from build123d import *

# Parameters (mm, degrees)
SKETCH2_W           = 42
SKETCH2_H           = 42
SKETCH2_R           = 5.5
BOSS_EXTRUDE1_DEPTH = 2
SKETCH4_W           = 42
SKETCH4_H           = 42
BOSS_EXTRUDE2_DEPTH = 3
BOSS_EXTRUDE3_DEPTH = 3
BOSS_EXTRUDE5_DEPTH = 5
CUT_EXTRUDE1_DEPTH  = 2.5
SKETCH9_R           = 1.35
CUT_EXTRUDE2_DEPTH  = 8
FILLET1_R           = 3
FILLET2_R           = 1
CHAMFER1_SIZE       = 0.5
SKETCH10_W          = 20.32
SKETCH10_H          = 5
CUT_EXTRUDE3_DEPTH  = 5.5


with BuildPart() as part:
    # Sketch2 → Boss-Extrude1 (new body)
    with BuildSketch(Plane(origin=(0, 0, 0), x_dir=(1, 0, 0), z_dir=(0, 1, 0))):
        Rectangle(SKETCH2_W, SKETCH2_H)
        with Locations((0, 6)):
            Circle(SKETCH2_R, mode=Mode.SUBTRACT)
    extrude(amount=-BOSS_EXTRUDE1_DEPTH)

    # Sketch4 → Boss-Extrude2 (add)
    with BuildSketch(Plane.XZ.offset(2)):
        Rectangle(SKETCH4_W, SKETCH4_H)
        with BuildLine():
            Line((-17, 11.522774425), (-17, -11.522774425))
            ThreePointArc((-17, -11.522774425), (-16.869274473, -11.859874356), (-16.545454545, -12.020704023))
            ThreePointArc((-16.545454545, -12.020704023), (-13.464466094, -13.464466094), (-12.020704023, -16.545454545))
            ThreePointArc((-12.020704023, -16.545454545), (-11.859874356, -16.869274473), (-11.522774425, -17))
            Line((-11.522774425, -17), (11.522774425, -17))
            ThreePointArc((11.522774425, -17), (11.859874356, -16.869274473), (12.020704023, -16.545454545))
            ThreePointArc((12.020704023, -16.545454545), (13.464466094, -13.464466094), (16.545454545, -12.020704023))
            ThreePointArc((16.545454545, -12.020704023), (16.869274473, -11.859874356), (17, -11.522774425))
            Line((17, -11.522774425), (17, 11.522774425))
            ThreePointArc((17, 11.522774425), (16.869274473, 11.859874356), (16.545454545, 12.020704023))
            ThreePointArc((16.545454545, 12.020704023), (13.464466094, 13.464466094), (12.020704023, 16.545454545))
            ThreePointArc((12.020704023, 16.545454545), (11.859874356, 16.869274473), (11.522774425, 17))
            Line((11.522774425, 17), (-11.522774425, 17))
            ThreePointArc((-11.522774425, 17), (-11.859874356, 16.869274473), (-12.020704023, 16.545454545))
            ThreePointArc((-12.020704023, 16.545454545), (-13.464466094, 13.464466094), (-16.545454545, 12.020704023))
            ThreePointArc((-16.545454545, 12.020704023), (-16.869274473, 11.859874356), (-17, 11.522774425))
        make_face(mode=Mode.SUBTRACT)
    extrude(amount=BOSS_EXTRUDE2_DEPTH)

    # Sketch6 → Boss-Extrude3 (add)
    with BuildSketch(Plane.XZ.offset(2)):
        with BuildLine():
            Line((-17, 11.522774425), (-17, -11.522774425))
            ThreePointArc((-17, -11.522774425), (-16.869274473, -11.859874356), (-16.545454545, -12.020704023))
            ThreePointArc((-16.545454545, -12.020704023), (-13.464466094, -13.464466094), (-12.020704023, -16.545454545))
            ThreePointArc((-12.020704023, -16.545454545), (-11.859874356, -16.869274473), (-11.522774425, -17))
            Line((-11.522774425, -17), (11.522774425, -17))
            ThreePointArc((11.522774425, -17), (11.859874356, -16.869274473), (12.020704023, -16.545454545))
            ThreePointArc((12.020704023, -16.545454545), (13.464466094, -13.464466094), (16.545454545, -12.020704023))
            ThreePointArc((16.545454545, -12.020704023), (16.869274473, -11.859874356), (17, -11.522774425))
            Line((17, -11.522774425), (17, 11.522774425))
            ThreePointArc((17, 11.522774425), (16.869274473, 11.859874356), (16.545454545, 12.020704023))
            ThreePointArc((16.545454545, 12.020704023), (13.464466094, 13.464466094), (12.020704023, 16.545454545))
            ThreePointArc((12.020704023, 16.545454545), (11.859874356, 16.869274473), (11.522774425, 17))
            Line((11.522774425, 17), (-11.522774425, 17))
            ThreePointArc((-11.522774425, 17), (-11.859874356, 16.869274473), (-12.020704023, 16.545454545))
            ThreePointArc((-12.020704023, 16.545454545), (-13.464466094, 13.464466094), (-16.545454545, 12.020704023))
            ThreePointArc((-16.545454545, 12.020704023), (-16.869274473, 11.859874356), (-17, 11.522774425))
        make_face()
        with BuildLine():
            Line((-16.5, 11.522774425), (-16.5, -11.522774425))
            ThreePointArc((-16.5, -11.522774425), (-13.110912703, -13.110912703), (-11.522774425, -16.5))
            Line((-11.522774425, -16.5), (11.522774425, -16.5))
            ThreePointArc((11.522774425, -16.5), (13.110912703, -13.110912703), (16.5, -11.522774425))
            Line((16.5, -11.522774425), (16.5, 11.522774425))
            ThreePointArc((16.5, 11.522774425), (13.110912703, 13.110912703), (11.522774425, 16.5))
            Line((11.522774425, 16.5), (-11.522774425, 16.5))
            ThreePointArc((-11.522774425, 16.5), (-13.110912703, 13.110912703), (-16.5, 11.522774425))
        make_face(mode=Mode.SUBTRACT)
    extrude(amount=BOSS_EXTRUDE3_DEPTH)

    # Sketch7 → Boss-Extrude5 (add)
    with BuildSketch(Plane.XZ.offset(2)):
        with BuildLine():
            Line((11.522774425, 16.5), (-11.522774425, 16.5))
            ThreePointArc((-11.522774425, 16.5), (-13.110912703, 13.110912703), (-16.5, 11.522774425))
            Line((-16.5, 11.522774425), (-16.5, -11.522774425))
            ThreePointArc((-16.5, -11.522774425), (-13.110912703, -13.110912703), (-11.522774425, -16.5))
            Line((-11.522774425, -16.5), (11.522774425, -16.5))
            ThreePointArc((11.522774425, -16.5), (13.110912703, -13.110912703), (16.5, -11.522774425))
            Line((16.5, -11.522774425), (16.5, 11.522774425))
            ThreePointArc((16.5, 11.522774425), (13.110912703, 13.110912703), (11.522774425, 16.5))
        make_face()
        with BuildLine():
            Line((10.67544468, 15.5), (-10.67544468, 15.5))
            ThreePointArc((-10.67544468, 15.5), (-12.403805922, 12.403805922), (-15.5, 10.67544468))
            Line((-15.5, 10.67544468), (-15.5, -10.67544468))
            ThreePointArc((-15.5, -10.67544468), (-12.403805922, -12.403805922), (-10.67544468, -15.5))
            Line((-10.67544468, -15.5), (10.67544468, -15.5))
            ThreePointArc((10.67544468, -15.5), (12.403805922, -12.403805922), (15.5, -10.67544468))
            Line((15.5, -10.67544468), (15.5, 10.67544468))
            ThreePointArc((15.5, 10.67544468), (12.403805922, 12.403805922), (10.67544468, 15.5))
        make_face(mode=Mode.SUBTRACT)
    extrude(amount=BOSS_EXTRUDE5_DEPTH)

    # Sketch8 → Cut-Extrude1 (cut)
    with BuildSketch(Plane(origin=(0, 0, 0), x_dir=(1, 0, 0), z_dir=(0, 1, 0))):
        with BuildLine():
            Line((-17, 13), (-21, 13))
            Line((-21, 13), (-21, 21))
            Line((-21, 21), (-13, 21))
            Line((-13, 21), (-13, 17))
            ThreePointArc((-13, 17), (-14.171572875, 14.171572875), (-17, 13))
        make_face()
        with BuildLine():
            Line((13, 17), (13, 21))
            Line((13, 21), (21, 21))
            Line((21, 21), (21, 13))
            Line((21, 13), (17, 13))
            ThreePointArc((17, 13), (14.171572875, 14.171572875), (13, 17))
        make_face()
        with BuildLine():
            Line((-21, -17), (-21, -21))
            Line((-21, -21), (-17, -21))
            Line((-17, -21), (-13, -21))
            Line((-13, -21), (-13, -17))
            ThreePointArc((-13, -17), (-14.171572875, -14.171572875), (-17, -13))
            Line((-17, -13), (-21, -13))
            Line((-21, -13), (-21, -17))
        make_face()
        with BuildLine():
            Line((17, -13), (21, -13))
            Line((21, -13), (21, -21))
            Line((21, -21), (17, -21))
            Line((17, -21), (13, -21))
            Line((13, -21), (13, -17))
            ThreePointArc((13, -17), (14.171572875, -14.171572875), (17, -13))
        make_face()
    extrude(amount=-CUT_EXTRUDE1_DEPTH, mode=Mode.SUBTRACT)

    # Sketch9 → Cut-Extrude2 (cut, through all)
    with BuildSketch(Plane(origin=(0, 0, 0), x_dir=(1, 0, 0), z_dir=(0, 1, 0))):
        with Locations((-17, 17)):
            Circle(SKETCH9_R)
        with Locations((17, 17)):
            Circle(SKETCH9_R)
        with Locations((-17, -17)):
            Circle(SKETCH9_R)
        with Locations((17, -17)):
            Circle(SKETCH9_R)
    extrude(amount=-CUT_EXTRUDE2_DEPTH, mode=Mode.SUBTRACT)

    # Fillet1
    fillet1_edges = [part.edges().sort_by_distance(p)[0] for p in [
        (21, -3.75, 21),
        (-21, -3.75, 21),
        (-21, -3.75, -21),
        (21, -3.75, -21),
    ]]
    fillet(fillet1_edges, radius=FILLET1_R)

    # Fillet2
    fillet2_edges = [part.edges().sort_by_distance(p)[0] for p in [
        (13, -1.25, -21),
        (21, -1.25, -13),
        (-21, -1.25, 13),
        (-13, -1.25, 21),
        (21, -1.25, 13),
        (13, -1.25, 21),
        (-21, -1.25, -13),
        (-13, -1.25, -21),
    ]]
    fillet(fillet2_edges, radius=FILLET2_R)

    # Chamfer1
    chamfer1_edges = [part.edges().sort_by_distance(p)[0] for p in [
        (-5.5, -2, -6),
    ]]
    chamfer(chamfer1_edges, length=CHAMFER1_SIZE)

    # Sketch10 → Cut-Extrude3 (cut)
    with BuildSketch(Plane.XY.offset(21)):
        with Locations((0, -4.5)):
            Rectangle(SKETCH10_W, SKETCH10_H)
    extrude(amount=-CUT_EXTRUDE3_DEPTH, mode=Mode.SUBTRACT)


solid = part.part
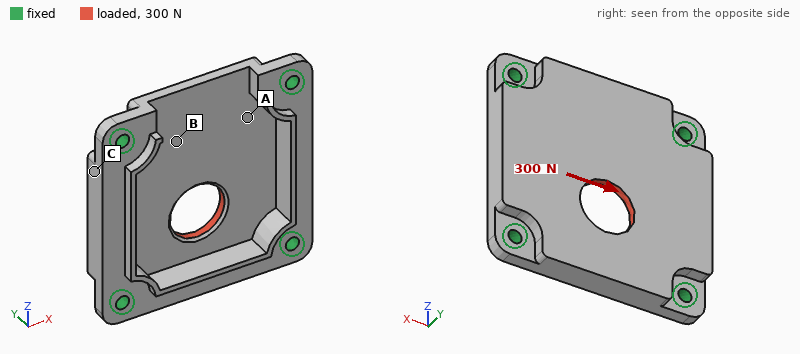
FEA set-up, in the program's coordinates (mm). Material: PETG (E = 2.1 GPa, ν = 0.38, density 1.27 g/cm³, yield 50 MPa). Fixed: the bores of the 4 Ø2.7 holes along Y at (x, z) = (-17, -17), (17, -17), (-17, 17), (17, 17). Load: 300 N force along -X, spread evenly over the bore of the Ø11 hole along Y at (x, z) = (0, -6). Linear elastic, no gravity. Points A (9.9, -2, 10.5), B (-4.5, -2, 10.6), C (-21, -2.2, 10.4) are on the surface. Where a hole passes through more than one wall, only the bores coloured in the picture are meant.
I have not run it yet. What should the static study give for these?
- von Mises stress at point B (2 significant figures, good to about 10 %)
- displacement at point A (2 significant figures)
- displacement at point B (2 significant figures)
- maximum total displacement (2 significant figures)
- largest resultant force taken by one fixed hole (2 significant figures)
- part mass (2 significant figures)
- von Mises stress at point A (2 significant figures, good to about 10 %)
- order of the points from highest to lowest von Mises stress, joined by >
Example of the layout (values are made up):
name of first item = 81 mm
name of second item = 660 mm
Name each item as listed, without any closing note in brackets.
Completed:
von Mises stress at point B = 2.1 MPa
displacement at point A = 43 µm
displacement at point B = 41 µm
maximum total displacement = 69 µm
largest resultant force taken by one fixed hole = 100 N
part mass = 6.5 g
von Mises stress at point A = 3.9 MPa
order of the points from highest to lowest von Mises stress, joined by > = A > B > C
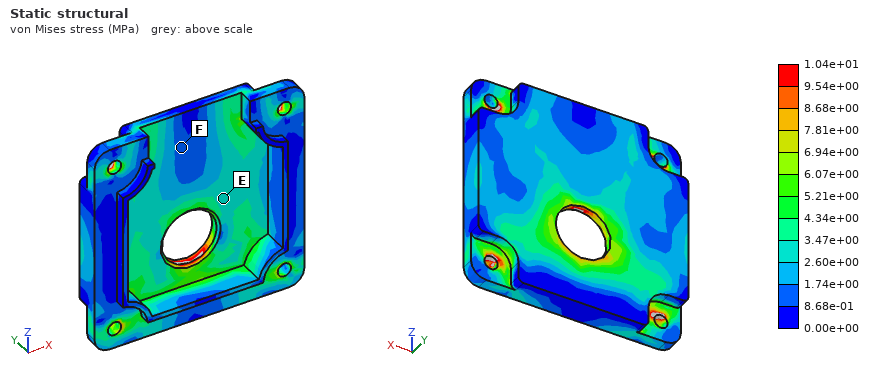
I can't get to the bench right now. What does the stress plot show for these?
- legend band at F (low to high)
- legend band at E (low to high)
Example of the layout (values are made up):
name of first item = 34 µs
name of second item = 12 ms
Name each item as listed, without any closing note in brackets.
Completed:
legend band at F = 8.68e-01 to 1.74e+00 MPa
legend band at E = 2.60e+00 to 3.47e+00 MPa
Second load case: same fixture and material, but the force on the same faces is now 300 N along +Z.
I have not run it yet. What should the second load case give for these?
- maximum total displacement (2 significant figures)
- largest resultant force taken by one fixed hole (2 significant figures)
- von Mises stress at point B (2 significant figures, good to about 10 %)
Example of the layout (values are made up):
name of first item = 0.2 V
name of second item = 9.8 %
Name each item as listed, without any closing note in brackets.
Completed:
maximum total displacement = 99 µm
largest resultant force taken by one fixed hole = 80 N
von Mises stress at point B = 3.1 MPa
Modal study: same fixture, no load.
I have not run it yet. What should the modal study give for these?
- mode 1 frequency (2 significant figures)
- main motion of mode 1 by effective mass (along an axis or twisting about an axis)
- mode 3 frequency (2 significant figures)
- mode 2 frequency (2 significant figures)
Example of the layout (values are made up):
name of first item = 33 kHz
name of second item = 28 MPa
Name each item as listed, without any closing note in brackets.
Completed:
mode 1 frequency = 2800 Hz
main motion of mode 1 by effective mass = along Y
mode 3 frequency = 4100 Hz
mode 2 frequency = 4000 Hz
